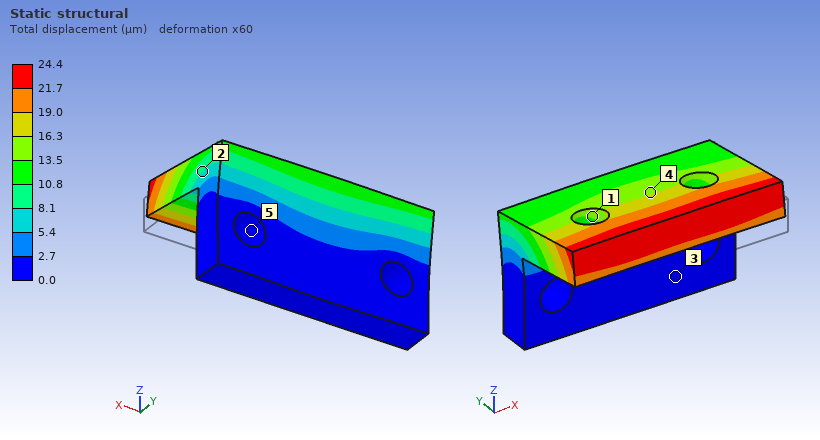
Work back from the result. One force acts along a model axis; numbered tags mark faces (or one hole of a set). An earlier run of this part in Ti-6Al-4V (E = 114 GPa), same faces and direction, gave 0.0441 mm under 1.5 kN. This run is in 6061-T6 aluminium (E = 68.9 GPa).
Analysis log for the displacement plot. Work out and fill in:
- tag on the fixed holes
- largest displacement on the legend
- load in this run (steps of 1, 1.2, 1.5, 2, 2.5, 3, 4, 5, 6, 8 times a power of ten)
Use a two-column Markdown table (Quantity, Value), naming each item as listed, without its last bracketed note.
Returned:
| Quantity | Value |
|---|---|
| tag on the fixed holes | 5 |
| largest displacement on the legend | 24.4 µm |
| load in this run | 500 N |
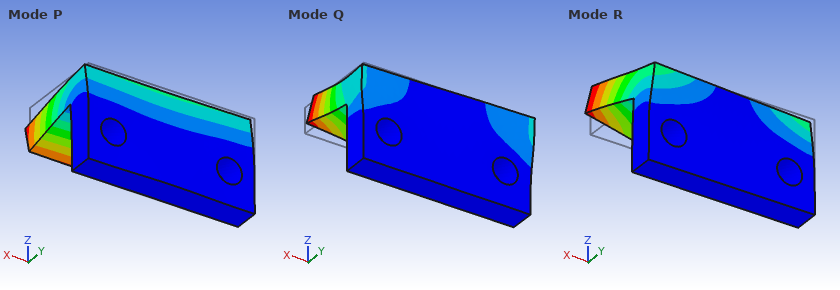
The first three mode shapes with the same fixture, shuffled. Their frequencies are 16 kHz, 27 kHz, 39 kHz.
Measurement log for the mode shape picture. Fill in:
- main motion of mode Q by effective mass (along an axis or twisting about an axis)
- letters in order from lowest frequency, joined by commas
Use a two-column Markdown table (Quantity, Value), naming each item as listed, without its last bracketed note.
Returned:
| Quantity | Value |
|---|---|
| main motion of mode Q by effective mass | along X |
| letters in order from lowest frequency, joined by commas | P, R, Q |
